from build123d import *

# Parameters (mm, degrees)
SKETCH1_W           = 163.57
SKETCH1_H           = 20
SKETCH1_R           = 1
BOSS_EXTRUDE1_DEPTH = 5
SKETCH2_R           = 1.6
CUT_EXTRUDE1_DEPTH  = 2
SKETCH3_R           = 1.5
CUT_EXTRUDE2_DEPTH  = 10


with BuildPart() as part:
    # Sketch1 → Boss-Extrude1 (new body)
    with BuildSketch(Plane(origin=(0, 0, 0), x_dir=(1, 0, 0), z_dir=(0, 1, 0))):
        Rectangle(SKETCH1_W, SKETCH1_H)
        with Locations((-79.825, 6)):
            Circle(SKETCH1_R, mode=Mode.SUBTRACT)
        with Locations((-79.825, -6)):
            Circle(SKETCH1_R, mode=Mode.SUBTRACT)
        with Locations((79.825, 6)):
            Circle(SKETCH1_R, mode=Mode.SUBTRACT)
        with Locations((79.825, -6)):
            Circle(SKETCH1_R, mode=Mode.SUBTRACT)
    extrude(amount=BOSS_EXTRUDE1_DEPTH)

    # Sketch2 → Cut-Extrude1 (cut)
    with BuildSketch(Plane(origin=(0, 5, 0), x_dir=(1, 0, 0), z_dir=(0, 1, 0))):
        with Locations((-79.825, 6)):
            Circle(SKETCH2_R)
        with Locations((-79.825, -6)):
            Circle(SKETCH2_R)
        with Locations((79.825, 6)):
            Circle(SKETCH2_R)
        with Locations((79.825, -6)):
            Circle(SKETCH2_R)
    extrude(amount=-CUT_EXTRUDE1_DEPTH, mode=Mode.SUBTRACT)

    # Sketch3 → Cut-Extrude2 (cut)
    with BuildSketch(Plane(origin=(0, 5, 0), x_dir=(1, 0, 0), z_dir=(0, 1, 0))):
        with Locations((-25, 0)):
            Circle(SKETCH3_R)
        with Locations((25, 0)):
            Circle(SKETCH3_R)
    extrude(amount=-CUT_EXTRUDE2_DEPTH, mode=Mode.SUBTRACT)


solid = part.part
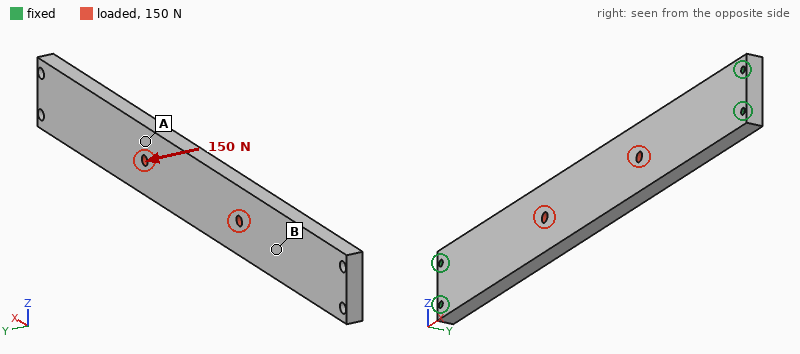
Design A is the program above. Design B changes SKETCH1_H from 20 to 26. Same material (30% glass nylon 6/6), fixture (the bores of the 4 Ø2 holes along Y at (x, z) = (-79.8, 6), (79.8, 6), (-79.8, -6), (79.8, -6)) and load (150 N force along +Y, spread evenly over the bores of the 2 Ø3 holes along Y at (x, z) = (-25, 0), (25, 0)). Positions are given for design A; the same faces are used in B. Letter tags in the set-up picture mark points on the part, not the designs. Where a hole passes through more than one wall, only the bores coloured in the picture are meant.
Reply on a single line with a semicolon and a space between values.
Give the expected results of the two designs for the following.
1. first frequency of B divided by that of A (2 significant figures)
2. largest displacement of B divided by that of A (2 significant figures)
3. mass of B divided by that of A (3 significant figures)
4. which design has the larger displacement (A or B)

0.97; 0.81; 1.30; A
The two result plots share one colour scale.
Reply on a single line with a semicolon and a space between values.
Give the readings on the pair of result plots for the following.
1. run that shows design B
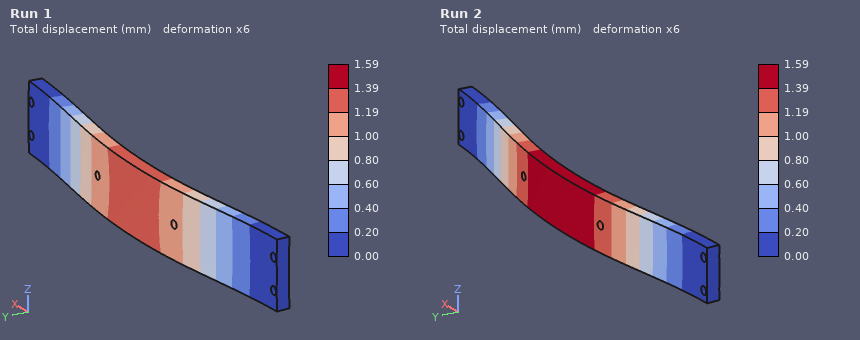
Run 1
